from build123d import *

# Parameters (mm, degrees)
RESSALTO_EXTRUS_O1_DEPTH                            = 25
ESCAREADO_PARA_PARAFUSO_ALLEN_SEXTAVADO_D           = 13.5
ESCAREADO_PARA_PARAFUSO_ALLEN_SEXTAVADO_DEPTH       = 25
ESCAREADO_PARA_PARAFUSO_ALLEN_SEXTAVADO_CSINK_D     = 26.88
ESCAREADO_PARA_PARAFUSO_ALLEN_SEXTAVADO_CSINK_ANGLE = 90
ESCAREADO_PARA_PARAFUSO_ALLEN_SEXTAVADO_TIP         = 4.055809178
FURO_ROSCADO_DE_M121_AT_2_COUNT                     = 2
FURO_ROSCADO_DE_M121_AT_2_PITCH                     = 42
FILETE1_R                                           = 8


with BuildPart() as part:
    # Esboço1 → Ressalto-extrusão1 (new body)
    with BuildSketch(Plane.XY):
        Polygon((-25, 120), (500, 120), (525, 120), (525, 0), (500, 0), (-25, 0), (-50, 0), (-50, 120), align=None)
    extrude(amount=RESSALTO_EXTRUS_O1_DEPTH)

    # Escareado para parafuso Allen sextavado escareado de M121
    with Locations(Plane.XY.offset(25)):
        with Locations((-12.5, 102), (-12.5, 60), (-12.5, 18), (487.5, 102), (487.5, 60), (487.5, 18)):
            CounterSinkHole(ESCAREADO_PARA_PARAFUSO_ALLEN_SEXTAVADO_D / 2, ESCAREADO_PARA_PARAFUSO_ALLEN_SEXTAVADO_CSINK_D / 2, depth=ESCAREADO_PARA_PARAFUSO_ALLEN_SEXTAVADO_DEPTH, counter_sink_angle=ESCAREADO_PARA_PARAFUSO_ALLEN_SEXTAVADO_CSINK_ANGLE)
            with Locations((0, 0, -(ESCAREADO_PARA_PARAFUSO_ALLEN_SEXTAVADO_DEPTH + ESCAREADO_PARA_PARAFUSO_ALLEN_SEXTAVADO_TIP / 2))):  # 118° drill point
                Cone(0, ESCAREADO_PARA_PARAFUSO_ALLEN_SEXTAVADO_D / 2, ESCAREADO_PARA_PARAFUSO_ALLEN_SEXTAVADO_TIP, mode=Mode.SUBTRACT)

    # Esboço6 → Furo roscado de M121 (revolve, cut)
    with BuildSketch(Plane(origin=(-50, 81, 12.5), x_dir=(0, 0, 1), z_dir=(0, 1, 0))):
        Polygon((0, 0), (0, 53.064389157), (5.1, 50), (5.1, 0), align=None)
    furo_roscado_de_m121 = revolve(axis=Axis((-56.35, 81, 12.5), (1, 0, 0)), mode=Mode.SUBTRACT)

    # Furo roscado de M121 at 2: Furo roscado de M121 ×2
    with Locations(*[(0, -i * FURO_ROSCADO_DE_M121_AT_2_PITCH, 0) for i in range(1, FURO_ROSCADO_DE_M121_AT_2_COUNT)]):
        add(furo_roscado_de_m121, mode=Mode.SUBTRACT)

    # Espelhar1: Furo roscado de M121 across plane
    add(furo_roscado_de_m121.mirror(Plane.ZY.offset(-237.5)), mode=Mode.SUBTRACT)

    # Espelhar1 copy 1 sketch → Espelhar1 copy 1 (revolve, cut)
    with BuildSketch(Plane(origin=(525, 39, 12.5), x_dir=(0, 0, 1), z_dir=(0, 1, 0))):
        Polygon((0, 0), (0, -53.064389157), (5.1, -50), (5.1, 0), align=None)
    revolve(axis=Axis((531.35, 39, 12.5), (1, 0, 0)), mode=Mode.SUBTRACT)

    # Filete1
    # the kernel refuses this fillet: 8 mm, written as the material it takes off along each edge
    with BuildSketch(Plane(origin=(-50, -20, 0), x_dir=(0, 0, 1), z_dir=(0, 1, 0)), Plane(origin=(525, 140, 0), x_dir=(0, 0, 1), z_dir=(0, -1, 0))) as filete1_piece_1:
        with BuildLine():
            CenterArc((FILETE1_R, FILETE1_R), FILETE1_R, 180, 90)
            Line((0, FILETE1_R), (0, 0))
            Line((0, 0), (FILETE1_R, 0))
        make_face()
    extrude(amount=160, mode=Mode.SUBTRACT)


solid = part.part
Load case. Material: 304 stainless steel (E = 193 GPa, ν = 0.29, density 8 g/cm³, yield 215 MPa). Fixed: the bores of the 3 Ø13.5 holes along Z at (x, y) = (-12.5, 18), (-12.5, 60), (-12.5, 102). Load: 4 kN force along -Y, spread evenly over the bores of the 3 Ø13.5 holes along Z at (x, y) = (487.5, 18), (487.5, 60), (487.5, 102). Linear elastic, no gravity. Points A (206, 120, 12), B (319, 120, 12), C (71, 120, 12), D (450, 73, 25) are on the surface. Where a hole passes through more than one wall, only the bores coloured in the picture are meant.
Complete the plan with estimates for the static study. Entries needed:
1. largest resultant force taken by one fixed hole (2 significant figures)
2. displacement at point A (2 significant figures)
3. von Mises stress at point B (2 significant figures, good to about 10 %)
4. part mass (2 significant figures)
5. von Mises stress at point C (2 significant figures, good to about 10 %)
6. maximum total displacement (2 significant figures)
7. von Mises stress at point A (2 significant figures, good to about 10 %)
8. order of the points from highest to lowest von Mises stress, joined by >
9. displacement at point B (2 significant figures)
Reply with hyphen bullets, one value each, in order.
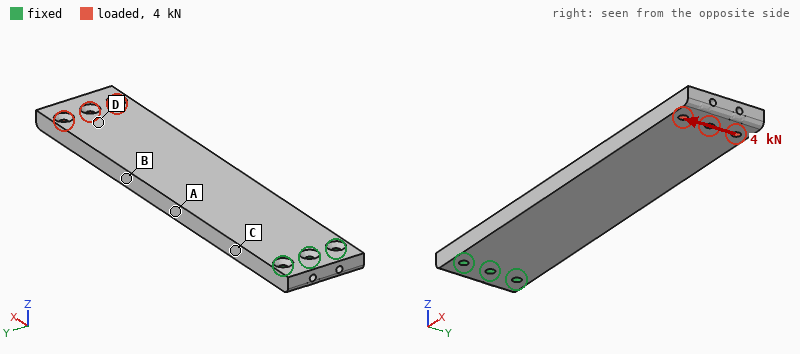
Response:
- 22 kN
- 0.074 mm
- 11 MPa
- 13 kg
- 28 MPa
- 0.29 mm
- 19 MPa
- C > A > B > D
- 0.14 mm
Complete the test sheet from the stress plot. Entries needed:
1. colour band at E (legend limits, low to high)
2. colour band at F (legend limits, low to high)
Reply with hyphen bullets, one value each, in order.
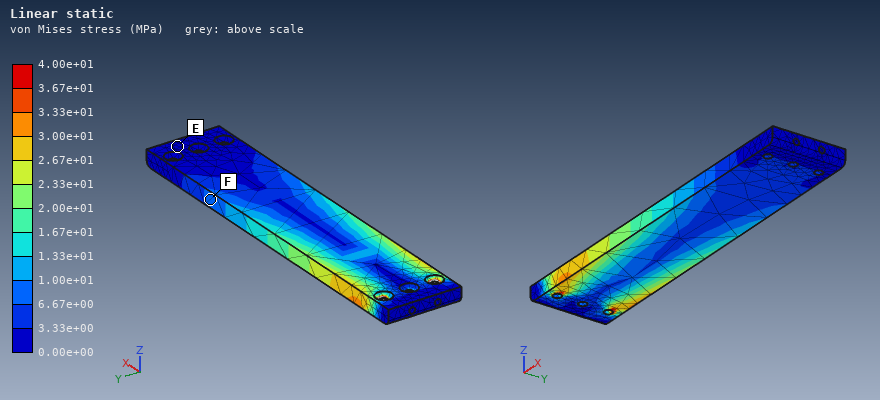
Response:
- 0.00e+00 to 3.33e+00 MPa
- 6.67e+00 to 1.00e+01 MPa
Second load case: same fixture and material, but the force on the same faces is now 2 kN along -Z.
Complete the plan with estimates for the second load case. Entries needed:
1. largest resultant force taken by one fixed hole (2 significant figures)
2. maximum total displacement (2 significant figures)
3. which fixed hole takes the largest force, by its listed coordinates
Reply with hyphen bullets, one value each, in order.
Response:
- 3.5 kN
- 3.2 mm
- (-12.5, 60)
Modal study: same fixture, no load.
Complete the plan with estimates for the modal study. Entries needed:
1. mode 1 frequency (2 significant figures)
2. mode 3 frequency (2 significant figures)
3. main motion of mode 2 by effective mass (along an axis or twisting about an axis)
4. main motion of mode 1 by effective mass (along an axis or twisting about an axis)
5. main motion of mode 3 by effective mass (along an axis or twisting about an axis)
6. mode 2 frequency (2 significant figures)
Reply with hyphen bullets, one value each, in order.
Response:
- 69 Hz
- 430 Hz
- along Y
- along Z
- along Z
- 320 Hz
